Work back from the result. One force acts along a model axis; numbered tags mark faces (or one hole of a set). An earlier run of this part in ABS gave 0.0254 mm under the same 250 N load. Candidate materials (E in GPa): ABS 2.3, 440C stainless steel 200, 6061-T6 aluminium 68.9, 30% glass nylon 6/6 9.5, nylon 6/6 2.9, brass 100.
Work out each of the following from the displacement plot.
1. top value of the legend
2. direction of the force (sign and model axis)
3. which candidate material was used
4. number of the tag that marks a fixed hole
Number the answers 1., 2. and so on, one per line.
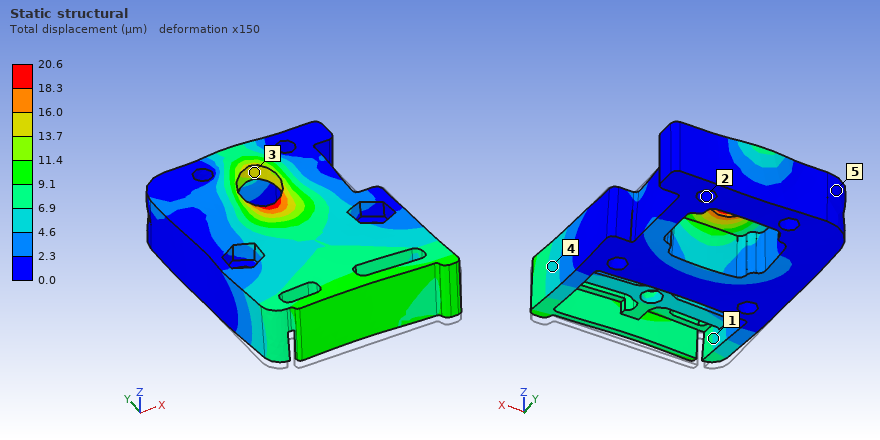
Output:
1. 20.6 µm
2. +Y
3. nylon 6/6
4. 2
